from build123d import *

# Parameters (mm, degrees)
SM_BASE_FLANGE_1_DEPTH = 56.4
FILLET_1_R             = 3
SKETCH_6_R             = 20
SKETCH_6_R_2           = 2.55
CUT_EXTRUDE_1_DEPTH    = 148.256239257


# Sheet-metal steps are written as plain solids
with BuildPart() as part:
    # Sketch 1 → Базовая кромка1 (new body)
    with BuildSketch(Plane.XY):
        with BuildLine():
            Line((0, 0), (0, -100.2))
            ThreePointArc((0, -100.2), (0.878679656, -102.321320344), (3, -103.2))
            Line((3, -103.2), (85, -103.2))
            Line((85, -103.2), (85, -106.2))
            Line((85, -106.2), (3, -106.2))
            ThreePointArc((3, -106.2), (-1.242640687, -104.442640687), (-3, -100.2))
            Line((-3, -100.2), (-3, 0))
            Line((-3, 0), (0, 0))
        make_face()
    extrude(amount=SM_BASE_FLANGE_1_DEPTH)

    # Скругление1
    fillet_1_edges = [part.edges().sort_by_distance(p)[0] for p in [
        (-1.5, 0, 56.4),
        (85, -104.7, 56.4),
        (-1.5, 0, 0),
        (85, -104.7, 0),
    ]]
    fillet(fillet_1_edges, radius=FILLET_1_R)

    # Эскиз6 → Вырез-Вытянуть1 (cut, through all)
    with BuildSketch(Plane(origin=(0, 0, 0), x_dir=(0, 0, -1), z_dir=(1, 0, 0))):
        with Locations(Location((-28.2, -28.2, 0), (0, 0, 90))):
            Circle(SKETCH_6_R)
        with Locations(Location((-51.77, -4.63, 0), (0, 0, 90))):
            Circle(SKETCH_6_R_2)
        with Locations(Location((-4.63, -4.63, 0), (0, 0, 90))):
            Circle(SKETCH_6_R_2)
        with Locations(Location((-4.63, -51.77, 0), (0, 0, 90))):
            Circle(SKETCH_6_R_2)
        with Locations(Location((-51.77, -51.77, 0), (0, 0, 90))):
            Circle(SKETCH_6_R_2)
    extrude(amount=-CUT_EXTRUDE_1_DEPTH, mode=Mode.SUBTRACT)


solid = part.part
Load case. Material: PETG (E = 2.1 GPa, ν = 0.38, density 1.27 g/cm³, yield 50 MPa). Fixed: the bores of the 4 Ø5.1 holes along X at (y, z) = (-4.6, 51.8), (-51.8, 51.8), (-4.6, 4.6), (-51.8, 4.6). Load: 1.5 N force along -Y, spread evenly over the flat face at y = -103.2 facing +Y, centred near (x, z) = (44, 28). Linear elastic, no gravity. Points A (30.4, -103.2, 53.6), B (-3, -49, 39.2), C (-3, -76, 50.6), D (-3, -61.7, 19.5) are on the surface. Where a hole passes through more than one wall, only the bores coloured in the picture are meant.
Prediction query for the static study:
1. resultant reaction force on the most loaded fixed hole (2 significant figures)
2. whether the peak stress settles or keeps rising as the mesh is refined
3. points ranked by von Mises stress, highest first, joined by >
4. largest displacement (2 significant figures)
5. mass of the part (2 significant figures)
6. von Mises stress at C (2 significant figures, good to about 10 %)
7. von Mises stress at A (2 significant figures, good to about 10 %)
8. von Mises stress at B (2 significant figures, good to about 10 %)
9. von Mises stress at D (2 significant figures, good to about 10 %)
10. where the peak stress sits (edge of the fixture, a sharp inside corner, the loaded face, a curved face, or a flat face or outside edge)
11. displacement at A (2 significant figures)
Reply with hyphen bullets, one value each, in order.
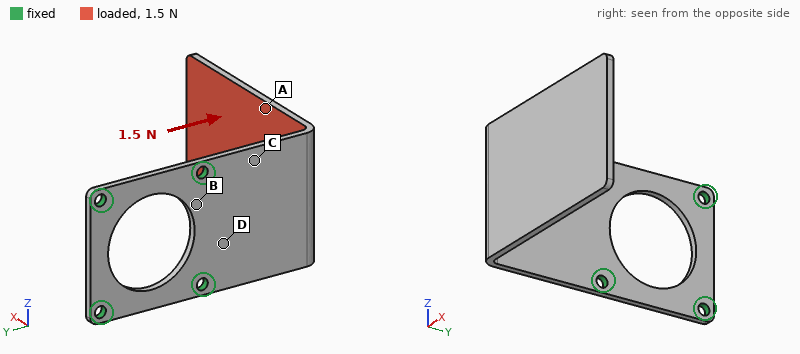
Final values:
- 0.78 N
- keeps rising
- C > D > B > A
- 1.6 mm
- 36 g
- 0.80 MPa
- 0.32 MPa
- 0.50 MPa
- 0.63 MPa
- edge of the fixture
- 0.61 mm
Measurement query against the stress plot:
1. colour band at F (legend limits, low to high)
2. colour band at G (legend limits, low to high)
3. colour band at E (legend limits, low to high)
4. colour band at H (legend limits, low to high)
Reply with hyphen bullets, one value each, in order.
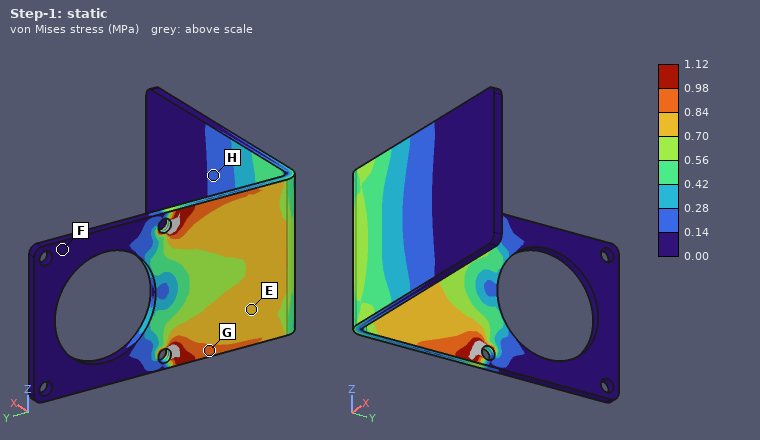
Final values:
- 0.00 to 0.14 MPa
- 0.84 to 0.98 MPa
- 0.70 to 0.84 MPa
- 0.14 to 0.28 MPa
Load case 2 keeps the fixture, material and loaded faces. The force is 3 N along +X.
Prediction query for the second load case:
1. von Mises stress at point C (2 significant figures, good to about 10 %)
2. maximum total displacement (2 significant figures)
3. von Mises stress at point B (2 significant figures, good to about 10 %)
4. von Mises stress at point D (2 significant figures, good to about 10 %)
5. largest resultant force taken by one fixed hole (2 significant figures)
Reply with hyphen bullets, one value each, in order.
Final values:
- 1.0 MPa
- 1.4 mm
- 1.0 MPa
- 1.1 MPa
- 1.6 N
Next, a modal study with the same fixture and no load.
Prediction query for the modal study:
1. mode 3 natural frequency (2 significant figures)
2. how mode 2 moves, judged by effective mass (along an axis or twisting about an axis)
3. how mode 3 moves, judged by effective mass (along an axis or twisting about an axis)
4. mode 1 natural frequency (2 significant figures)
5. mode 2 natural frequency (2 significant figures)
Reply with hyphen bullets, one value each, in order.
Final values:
- 130 Hz
- along Z
- along X
- 42 Hz
- 76 Hz
